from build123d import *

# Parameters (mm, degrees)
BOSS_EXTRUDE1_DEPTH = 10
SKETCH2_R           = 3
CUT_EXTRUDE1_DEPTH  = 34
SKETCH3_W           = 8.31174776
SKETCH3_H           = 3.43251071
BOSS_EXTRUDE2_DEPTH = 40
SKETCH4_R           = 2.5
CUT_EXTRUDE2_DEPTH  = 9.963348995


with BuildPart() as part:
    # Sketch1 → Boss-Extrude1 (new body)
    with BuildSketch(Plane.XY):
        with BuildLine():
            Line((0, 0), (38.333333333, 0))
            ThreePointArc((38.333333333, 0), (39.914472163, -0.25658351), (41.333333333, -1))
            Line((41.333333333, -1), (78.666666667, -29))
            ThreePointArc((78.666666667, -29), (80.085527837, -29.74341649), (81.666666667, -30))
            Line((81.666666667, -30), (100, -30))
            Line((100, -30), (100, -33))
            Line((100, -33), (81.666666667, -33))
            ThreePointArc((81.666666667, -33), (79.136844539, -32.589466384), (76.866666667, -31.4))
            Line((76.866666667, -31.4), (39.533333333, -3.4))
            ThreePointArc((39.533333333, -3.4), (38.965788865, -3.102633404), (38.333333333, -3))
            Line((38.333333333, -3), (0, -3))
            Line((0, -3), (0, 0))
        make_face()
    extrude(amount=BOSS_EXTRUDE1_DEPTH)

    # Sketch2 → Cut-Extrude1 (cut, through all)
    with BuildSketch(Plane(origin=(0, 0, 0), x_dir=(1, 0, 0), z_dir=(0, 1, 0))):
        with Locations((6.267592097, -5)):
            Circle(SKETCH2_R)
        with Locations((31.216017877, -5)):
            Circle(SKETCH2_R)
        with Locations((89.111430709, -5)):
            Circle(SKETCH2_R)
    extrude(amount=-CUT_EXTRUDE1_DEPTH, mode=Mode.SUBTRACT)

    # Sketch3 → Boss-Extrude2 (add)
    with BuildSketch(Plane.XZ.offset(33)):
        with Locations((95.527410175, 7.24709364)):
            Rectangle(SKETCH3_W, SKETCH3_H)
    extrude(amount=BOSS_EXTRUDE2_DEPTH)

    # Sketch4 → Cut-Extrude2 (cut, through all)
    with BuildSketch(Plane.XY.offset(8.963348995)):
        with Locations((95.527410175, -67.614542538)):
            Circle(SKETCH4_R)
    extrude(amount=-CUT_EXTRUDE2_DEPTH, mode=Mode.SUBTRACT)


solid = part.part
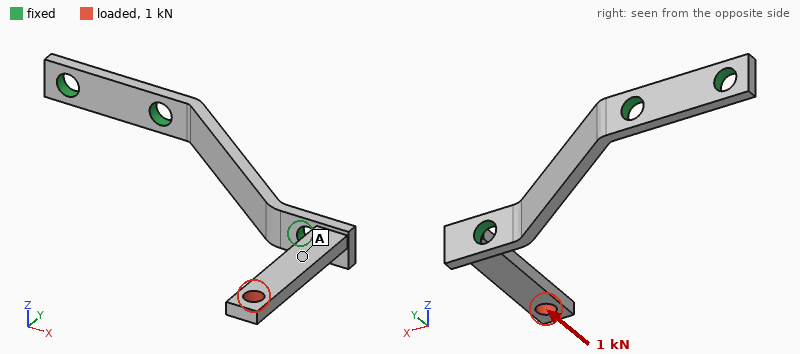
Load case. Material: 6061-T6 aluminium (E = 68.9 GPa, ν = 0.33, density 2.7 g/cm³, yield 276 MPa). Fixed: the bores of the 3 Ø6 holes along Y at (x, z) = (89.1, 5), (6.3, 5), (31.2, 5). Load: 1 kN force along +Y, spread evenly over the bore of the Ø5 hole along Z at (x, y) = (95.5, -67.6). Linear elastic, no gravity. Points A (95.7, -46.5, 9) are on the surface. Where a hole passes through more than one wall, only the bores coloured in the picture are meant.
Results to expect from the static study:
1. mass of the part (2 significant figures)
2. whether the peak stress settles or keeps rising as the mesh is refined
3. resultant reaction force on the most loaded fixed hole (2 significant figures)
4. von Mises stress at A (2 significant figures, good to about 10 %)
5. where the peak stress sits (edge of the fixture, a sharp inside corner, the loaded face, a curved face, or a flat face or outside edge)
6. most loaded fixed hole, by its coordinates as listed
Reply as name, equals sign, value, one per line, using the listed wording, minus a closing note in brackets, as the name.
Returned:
mass of the part = 11 g
whether the peak stress settles or keeps rising as the mesh is refined = keeps rising
resultant reaction force on the most loaded fixed hole = 1.0 kN
von Mises stress at A = 35 MPa
where the peak stress sits = edge of the fixture
most loaded fixed hole, by its coordinates as listed = (89.1, 5)
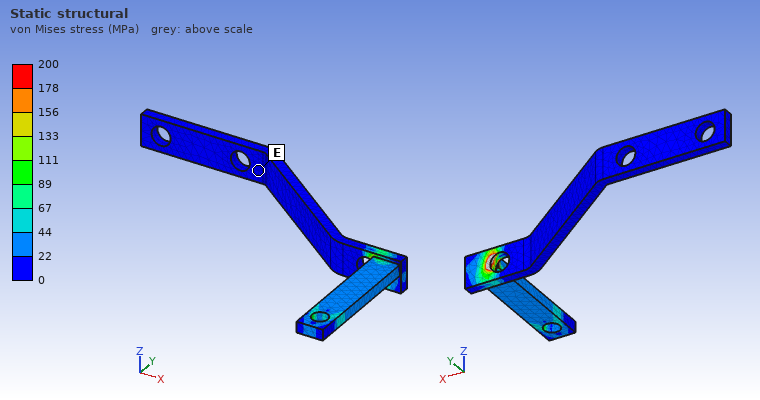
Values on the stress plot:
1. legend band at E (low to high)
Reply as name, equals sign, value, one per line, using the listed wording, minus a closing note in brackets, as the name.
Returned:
legend band at E = 0 to 22 MPa
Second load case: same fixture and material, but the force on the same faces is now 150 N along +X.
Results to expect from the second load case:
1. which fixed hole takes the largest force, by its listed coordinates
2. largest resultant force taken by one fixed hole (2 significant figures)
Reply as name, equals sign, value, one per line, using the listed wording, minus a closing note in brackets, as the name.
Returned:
which fixed hole takes the largest force, by its listed coordinates = (89.1, 5)
largest resultant force taken by one fixed hole = 150 N
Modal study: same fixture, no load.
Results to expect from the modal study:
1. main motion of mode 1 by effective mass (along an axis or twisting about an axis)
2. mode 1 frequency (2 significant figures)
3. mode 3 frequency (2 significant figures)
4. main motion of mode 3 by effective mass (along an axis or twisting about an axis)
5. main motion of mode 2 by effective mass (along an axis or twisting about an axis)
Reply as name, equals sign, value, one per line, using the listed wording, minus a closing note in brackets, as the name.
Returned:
main motion of mode 1 by effective mass = along Z
mode 1 frequency = 1600 Hz
mode 3 frequency = 4000 Hz
main motion of mode 3 by effective mass = along Y
main motion of mode 2 by effective mass = along X
